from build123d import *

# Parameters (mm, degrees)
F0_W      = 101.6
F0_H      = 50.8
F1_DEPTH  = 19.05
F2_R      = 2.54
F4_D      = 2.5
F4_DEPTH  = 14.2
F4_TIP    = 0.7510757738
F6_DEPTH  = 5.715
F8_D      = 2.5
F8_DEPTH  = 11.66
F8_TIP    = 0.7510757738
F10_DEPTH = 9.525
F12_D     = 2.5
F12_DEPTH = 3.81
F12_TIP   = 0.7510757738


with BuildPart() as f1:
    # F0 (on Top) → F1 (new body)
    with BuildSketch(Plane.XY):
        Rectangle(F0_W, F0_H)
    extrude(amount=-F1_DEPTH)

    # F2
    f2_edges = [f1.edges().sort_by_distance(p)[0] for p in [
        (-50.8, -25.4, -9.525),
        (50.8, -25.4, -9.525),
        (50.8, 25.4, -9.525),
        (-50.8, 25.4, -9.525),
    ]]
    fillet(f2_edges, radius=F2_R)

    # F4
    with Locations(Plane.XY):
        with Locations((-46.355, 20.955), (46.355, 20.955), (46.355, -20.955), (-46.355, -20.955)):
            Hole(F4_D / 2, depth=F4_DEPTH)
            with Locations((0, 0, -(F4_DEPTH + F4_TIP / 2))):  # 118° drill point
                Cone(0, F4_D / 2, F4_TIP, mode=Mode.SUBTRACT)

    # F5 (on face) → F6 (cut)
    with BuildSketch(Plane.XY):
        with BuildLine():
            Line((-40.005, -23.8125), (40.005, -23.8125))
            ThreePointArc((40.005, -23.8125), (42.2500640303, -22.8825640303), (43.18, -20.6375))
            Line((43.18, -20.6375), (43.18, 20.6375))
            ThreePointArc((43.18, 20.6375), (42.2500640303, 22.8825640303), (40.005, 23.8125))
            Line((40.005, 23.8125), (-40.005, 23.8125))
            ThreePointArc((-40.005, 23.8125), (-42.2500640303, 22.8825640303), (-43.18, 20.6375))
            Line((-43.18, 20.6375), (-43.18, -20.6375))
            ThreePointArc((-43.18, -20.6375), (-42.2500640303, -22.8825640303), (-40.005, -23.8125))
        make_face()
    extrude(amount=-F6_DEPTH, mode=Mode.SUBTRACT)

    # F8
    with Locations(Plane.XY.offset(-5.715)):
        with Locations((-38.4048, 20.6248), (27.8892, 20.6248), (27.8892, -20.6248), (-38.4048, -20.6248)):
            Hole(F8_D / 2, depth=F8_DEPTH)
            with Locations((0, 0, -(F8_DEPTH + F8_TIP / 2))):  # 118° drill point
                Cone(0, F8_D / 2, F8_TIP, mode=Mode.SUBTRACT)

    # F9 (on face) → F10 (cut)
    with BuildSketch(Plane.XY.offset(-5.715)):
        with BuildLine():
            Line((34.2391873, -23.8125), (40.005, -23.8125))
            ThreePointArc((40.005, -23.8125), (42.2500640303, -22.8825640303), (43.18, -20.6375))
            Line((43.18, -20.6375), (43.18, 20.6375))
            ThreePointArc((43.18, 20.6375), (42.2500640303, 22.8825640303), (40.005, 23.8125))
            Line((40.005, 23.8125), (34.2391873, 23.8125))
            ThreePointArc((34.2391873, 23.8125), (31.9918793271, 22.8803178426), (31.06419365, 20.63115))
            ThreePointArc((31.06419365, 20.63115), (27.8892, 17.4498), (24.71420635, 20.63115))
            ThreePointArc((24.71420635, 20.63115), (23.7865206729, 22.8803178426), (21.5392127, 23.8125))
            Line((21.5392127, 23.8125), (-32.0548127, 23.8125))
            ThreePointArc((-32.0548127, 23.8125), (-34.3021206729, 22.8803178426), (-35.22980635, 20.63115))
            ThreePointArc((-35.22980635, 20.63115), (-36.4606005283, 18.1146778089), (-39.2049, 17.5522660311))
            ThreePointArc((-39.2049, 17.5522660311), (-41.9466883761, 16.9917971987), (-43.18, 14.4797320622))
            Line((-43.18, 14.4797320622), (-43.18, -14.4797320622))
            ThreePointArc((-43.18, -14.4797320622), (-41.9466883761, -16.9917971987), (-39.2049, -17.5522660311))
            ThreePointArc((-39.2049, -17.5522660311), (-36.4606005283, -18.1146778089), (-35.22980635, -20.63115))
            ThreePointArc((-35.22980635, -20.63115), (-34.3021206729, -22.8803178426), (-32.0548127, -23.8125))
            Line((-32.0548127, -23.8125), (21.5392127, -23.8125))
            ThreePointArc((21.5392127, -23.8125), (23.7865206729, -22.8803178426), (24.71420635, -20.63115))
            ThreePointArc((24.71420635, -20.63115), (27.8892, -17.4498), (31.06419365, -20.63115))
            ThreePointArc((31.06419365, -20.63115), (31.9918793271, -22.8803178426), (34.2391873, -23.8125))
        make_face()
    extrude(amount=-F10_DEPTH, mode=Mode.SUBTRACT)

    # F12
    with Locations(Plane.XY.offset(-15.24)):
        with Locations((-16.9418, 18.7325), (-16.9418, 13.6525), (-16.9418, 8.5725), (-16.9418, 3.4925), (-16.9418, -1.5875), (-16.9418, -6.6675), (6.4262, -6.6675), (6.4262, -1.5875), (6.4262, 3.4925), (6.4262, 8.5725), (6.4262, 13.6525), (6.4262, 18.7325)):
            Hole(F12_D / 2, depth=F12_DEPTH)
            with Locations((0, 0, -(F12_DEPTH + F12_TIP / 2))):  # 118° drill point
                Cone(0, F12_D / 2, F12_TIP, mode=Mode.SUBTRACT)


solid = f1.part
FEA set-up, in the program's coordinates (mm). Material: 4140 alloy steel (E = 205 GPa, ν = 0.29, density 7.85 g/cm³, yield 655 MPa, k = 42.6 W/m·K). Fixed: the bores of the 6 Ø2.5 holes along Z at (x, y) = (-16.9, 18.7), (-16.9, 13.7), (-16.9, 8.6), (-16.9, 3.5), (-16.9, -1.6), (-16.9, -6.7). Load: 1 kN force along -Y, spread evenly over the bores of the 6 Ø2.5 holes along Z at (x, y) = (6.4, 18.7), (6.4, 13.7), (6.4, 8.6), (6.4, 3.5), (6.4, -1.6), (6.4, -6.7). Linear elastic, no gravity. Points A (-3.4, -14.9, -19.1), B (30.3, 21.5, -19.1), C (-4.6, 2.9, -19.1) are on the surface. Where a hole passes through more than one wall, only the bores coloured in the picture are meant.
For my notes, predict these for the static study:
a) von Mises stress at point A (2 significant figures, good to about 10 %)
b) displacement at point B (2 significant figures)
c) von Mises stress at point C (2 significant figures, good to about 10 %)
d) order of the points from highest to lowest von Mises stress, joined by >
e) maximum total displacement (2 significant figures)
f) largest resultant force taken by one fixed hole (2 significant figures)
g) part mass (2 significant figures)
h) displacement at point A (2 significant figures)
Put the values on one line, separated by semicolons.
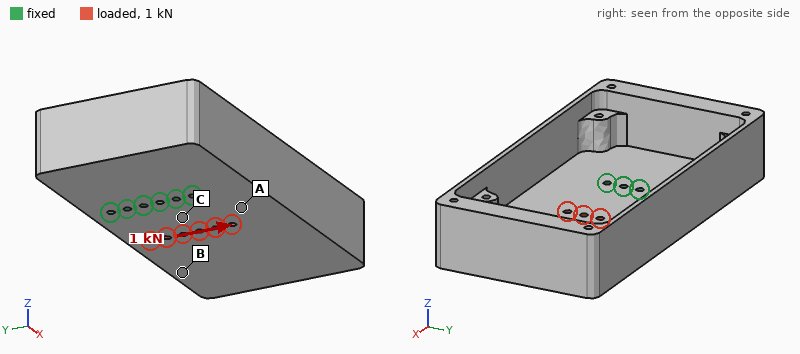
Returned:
5.2 MPa; 5.3 µm; 15 MPa; C > A > B; 7.8 µm; 760 N; 290 g; 2.3 µm
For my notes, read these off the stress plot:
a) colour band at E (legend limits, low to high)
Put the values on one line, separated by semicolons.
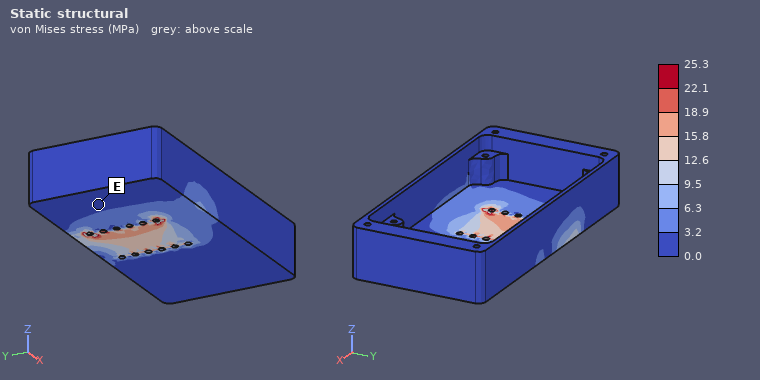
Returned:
0.0 to 3.2 MPa
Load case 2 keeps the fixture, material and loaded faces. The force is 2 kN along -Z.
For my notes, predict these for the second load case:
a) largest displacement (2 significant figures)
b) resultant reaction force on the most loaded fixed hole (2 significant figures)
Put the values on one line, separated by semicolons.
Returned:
0.28 mm; 870 N
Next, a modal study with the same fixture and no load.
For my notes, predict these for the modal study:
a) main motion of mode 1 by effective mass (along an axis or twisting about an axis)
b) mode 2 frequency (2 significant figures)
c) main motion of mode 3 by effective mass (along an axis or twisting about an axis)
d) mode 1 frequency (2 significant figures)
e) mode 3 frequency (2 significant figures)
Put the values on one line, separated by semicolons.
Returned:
along Z; 1800 Hz; along Z; 730 Hz; 2600 Hz
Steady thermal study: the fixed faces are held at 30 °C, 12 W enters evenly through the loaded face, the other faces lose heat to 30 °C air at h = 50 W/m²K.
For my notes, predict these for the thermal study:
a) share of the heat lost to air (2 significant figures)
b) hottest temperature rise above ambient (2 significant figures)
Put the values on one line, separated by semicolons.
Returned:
53 %; 24 K
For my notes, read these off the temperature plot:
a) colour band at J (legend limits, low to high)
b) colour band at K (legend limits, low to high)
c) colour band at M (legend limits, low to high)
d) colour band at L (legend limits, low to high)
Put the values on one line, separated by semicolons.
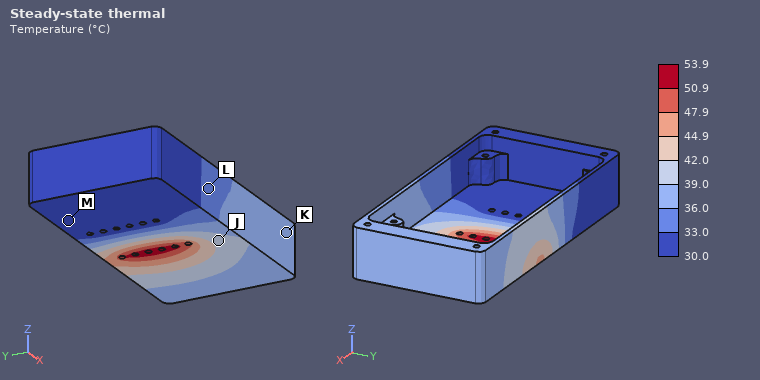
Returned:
39.0 to 42.0 °C; 36.0 to 39.0 °C; 30.0 to 33.0 °C; 33.0 to 36.0 °C
